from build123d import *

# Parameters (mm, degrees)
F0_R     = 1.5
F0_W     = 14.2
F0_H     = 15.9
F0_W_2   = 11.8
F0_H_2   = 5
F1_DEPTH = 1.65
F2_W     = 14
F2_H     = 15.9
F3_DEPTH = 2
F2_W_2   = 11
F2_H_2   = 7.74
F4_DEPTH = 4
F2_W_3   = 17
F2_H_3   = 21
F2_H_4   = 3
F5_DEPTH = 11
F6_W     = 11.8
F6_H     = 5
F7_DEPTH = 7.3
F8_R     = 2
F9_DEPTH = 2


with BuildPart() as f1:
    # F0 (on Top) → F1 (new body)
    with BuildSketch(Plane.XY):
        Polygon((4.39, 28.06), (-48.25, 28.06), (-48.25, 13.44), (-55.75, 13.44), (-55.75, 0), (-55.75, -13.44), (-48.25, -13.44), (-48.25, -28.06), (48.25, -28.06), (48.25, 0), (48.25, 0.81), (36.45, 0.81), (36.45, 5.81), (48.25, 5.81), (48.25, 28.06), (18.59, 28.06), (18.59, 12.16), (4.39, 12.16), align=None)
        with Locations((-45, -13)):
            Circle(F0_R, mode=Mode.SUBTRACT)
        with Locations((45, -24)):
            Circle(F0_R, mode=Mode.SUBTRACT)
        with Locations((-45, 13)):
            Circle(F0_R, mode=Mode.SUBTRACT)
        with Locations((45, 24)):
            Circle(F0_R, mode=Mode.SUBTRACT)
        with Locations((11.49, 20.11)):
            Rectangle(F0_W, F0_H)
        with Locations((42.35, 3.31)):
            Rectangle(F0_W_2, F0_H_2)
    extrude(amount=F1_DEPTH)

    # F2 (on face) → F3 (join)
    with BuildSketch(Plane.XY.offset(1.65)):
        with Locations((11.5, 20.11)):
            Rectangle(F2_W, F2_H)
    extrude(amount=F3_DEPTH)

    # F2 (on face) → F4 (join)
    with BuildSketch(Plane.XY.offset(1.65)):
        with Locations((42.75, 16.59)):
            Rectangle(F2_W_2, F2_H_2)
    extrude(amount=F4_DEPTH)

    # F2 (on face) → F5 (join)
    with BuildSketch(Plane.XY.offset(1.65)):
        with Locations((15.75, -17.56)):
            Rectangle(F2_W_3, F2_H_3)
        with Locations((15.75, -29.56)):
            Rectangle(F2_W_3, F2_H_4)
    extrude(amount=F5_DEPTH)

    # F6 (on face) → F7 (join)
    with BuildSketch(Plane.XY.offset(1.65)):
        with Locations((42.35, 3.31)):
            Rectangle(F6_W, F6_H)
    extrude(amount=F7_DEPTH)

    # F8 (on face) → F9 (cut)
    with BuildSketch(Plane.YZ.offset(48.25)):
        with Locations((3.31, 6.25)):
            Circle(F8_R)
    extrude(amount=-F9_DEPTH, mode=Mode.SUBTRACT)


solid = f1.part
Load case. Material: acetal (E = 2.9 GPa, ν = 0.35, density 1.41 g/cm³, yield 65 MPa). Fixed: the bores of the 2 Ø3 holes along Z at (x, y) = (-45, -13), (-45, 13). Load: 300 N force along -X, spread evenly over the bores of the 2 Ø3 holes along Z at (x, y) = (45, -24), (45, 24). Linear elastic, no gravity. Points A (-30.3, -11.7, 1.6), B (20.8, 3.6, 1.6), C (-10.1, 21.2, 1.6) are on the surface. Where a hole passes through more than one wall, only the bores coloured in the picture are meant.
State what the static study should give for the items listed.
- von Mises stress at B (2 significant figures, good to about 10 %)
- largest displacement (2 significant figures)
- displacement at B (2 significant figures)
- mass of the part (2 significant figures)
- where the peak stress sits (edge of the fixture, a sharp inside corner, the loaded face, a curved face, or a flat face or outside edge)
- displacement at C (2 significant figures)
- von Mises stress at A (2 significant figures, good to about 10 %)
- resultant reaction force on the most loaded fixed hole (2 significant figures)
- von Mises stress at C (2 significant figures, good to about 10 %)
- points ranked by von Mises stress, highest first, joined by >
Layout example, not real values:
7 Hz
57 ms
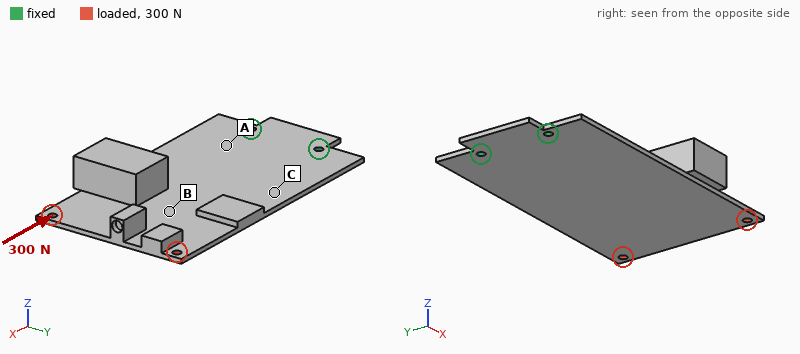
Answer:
1.2 MPa
0.28 mm
0.095 mm
21 g
the loaded face
0.058 mm
4.3 MPa
150 N
3.2 MPa
A > C > B
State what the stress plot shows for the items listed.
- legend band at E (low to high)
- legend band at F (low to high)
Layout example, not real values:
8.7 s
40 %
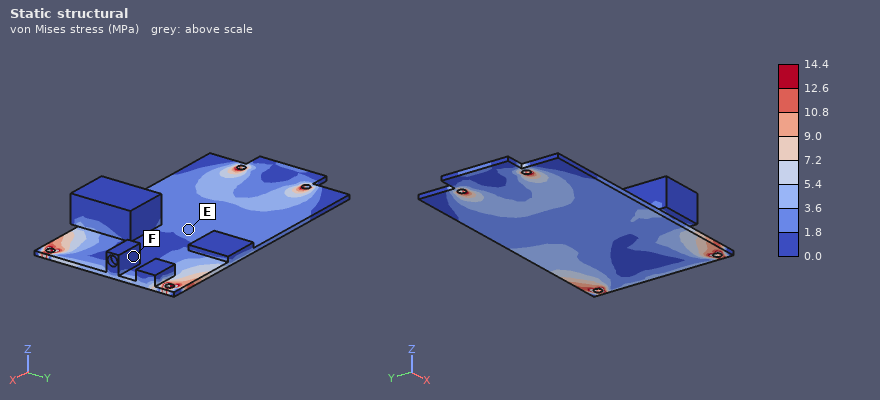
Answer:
1.8 to 3.6 MPa
0.0 to 1.8 MPa
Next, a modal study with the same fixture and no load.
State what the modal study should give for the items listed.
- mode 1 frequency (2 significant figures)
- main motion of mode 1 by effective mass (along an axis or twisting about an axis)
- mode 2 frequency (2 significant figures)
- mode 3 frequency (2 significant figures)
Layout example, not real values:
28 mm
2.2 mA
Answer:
31 Hz
along Z
110 Hz
250 Hz
